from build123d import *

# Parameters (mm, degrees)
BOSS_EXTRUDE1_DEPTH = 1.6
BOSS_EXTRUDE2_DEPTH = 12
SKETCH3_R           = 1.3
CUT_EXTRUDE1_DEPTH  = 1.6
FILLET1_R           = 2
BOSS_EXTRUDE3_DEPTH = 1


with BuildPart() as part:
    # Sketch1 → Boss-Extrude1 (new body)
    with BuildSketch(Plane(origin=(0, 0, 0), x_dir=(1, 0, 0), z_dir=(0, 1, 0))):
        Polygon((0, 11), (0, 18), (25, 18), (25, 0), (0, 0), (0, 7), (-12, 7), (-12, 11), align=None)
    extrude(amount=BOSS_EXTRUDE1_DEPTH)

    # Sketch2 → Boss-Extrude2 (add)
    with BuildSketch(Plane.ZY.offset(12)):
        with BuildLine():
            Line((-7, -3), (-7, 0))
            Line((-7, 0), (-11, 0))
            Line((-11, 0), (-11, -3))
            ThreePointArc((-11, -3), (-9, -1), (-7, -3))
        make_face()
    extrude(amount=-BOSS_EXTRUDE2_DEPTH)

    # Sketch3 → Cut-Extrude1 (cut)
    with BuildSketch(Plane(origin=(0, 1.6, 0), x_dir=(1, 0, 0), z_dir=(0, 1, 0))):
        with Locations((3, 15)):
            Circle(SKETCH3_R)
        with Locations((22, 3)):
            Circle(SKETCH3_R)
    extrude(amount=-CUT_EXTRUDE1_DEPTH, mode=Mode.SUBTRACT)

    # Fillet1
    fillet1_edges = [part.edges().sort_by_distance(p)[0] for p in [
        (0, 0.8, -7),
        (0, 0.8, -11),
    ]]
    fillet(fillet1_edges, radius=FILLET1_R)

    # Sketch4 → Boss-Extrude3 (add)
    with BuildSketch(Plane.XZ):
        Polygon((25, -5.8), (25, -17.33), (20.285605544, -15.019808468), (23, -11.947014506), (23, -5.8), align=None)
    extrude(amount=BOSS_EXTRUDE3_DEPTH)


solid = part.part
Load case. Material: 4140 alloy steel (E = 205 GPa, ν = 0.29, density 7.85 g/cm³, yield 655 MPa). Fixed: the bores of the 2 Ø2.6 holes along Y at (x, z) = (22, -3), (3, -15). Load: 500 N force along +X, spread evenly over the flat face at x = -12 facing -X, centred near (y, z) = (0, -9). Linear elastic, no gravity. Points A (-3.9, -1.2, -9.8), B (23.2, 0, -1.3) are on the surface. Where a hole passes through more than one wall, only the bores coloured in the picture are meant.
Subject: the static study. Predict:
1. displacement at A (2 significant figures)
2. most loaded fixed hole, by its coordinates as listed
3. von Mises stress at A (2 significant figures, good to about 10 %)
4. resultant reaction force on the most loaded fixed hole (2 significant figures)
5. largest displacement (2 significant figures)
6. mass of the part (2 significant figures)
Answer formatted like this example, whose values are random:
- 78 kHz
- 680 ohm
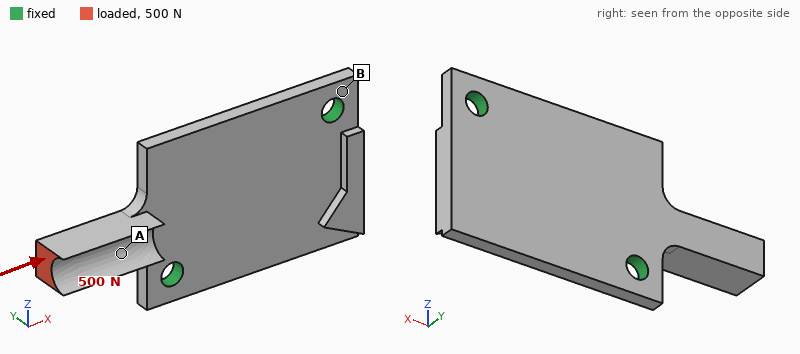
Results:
- 21 µm
- (3, -15)
- 44 MPa
- 310 N
- 53 µm
- 6.9 g
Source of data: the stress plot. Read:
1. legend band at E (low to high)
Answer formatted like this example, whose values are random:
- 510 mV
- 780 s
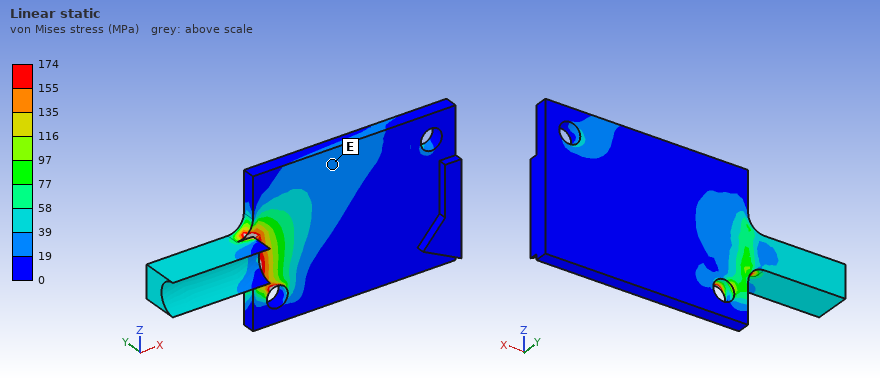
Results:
- 19 to 39 MPa
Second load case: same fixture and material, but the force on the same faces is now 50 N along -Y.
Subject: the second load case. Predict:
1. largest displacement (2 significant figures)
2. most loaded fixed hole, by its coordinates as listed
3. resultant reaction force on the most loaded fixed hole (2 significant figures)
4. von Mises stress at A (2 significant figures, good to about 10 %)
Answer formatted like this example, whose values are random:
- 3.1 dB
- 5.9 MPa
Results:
- 0.11 mm
- (3, -15)
- 67 N
- 51 MPa
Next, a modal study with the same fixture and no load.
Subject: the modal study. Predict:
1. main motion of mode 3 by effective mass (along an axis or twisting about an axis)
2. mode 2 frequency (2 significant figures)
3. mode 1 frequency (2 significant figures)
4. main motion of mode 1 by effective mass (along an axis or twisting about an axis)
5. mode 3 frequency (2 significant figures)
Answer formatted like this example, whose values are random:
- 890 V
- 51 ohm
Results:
- along Y
- 7900 Hz
- 5100 Hz
- along Y
- 9700 Hz
